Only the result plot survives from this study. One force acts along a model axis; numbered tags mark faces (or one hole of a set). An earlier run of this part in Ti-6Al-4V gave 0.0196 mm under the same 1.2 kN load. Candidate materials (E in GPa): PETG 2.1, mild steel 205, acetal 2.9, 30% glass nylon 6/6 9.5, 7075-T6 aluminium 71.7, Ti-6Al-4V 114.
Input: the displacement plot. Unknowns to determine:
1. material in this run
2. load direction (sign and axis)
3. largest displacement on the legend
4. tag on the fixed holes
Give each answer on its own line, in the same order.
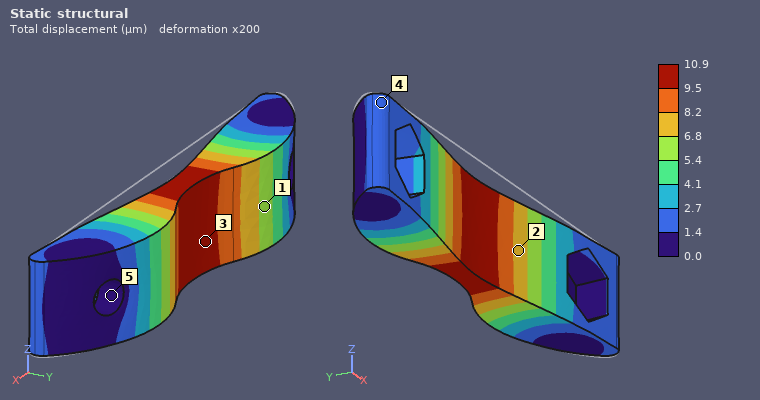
mild steel
+Y
10.9 µm
5
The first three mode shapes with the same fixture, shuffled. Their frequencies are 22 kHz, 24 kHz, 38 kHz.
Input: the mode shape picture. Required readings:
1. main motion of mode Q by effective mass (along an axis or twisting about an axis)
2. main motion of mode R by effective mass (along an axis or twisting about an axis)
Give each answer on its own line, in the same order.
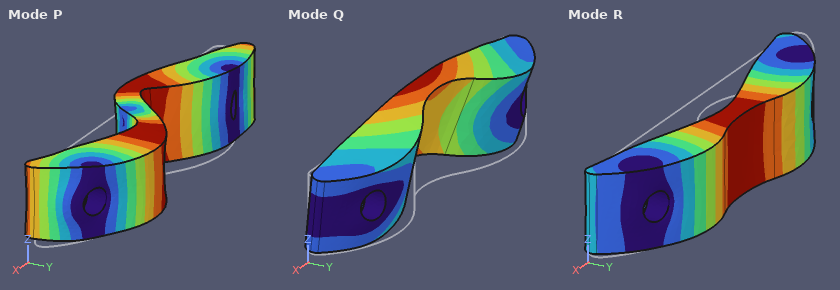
along Z
along Y
